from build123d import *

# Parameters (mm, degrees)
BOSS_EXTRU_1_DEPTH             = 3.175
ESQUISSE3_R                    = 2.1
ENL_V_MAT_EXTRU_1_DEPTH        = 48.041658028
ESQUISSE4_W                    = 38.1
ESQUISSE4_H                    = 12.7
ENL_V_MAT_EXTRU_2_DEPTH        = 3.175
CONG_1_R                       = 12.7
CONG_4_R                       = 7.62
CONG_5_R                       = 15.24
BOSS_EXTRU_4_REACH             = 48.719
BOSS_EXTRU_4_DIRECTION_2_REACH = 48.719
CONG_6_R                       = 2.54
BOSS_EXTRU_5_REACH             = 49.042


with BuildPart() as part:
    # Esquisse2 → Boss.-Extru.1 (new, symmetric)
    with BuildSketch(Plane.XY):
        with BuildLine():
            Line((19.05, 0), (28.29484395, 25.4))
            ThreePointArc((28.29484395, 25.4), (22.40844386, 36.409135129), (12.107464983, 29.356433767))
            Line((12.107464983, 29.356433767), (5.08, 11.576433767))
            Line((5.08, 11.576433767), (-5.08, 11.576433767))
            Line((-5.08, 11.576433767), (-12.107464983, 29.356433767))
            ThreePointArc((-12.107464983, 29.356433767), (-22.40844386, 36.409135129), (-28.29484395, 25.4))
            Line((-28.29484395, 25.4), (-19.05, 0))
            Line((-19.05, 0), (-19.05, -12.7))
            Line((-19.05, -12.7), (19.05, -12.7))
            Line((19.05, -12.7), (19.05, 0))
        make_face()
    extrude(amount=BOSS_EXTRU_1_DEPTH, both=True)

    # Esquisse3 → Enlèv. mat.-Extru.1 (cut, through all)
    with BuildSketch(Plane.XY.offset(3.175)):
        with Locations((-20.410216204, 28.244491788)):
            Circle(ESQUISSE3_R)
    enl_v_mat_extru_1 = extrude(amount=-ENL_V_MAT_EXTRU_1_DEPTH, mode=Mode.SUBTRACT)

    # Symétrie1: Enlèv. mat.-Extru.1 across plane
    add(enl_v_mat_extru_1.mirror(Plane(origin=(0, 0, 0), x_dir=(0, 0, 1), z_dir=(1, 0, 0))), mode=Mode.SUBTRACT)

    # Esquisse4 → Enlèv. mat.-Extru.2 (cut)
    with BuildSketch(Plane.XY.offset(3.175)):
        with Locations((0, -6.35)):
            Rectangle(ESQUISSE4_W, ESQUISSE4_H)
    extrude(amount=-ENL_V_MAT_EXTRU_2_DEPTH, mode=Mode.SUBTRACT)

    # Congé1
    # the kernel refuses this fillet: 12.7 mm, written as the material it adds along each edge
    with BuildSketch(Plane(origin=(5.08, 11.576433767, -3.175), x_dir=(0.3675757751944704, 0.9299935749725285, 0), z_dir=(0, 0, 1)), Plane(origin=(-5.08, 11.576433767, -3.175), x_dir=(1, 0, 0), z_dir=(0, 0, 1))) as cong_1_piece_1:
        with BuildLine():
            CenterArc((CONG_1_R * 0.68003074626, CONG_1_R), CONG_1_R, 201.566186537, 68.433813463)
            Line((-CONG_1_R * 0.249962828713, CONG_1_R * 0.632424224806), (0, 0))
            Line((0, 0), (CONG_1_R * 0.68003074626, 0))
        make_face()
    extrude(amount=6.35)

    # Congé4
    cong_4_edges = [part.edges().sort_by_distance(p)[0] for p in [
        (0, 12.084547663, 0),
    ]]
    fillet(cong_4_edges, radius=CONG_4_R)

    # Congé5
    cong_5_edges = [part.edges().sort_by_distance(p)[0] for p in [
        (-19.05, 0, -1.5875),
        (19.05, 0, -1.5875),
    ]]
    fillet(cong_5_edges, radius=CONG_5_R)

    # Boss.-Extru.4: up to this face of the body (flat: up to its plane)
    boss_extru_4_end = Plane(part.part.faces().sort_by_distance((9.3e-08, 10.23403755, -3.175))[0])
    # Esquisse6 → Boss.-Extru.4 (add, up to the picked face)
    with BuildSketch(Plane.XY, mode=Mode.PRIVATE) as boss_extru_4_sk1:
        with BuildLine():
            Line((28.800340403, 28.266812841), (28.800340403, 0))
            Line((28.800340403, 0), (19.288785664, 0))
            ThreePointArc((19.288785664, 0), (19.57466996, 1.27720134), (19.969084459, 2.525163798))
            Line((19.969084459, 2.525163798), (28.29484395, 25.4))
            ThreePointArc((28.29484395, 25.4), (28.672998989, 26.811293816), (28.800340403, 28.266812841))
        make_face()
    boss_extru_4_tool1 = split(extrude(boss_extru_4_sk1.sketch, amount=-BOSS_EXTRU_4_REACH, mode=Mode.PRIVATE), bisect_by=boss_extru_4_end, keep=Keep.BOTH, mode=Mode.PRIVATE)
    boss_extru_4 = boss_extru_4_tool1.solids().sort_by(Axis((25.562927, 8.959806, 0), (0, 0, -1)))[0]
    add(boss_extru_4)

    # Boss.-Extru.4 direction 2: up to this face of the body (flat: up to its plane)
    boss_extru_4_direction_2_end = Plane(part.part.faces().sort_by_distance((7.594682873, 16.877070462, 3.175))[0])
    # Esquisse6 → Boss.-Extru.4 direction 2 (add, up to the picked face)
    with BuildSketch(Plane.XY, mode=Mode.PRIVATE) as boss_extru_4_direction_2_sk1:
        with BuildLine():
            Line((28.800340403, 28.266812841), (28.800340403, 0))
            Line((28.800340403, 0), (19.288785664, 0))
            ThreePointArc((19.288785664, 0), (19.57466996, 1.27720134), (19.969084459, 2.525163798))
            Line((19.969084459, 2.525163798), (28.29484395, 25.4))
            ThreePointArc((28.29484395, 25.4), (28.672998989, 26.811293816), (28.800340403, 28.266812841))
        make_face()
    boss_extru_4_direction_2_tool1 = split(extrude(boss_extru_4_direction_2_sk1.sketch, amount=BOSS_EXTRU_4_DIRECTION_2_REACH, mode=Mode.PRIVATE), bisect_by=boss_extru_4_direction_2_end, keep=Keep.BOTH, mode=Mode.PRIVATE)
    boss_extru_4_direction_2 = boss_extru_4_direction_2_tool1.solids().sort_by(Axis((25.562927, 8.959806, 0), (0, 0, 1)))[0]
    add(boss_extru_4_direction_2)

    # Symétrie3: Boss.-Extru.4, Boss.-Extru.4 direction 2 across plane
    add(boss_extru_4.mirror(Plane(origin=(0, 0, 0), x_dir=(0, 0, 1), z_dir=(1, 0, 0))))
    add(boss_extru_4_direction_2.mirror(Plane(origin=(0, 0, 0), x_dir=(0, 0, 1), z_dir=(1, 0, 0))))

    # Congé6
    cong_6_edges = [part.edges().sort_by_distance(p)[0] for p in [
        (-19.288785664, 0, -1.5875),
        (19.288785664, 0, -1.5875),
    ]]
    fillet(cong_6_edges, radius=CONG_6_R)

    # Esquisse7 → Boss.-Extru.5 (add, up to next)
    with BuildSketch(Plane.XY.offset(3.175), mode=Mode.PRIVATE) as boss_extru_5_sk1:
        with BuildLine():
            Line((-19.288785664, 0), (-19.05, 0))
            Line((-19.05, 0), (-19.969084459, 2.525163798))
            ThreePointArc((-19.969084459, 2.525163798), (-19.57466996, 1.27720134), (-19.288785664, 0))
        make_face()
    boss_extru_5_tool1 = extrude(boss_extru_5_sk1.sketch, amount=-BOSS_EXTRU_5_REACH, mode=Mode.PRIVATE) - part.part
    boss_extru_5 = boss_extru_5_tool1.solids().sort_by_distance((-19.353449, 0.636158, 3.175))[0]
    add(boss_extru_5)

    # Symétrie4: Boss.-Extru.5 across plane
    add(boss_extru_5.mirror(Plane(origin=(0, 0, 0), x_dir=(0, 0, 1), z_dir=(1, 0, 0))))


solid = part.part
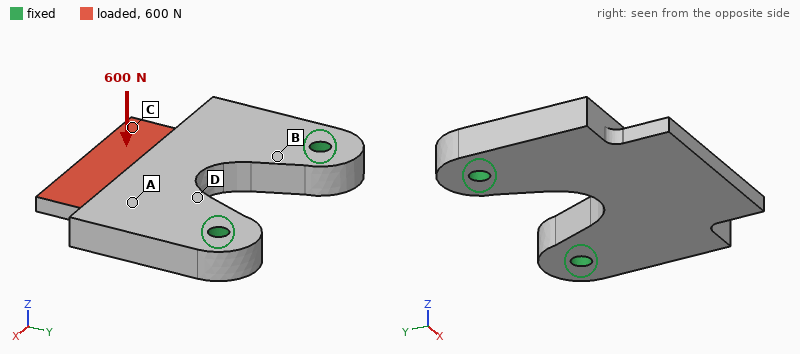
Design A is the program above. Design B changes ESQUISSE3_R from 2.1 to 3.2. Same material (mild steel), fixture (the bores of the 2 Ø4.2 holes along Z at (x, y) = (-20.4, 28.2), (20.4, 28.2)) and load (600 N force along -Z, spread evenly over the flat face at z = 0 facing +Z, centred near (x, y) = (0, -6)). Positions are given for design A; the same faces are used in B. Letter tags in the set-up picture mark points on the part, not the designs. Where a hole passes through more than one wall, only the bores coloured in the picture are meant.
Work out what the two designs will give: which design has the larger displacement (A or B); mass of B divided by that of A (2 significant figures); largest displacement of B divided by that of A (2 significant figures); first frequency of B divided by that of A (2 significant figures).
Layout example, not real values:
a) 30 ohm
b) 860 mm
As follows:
a) A
b) 0.98
c) 0.89
d) 1.1
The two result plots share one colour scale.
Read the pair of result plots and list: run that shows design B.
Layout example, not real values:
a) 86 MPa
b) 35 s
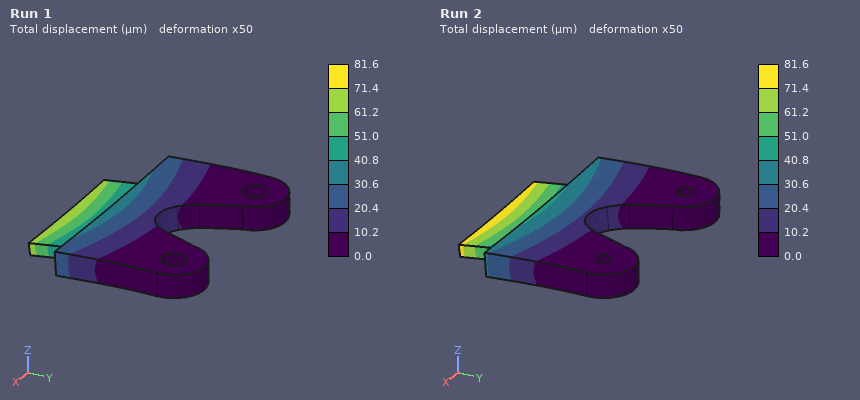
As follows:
a) Run 1
